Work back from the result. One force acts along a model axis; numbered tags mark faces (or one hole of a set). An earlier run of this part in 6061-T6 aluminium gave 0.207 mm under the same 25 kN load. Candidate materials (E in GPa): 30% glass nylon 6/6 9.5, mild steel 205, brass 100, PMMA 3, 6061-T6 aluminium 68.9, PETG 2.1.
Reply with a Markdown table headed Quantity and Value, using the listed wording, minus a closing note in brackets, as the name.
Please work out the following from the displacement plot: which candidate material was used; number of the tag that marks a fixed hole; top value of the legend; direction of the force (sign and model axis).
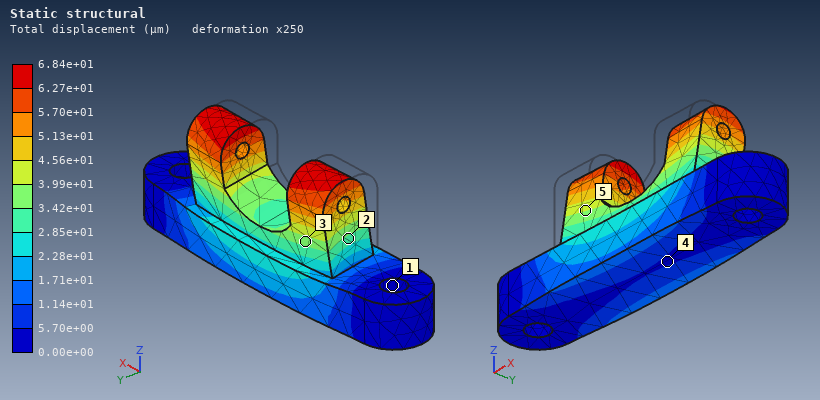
| Quantity | Value |
|---|---|
| which candidate material was used | mild steel |
| number of the tag that marks a fixed hole | 1 |
| top value of the legend | 6.84e+01 µm |
| direction of the force | +Y |
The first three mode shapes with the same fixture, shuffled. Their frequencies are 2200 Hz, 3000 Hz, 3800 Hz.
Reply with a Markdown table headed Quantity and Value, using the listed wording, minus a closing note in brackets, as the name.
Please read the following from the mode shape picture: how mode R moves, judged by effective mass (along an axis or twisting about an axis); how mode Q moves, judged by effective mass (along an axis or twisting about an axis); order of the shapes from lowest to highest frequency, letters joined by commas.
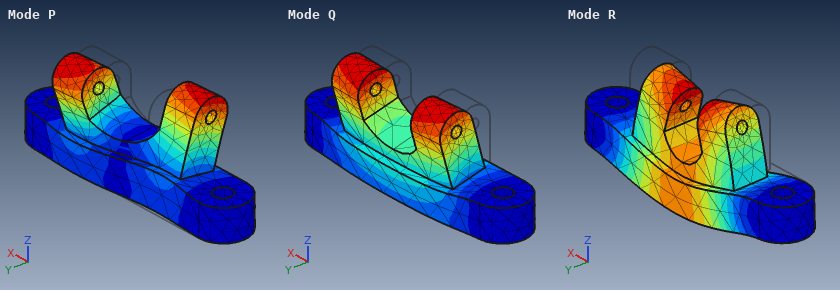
| Quantity | Value |
|---|---|
| how mode R moves, judged by effective mass | along Z |
| how mode Q moves, judged by effective mass | along Y |
| order of the shapes from lowest to highest frequency, letters joined by commas | Q, R, P |
